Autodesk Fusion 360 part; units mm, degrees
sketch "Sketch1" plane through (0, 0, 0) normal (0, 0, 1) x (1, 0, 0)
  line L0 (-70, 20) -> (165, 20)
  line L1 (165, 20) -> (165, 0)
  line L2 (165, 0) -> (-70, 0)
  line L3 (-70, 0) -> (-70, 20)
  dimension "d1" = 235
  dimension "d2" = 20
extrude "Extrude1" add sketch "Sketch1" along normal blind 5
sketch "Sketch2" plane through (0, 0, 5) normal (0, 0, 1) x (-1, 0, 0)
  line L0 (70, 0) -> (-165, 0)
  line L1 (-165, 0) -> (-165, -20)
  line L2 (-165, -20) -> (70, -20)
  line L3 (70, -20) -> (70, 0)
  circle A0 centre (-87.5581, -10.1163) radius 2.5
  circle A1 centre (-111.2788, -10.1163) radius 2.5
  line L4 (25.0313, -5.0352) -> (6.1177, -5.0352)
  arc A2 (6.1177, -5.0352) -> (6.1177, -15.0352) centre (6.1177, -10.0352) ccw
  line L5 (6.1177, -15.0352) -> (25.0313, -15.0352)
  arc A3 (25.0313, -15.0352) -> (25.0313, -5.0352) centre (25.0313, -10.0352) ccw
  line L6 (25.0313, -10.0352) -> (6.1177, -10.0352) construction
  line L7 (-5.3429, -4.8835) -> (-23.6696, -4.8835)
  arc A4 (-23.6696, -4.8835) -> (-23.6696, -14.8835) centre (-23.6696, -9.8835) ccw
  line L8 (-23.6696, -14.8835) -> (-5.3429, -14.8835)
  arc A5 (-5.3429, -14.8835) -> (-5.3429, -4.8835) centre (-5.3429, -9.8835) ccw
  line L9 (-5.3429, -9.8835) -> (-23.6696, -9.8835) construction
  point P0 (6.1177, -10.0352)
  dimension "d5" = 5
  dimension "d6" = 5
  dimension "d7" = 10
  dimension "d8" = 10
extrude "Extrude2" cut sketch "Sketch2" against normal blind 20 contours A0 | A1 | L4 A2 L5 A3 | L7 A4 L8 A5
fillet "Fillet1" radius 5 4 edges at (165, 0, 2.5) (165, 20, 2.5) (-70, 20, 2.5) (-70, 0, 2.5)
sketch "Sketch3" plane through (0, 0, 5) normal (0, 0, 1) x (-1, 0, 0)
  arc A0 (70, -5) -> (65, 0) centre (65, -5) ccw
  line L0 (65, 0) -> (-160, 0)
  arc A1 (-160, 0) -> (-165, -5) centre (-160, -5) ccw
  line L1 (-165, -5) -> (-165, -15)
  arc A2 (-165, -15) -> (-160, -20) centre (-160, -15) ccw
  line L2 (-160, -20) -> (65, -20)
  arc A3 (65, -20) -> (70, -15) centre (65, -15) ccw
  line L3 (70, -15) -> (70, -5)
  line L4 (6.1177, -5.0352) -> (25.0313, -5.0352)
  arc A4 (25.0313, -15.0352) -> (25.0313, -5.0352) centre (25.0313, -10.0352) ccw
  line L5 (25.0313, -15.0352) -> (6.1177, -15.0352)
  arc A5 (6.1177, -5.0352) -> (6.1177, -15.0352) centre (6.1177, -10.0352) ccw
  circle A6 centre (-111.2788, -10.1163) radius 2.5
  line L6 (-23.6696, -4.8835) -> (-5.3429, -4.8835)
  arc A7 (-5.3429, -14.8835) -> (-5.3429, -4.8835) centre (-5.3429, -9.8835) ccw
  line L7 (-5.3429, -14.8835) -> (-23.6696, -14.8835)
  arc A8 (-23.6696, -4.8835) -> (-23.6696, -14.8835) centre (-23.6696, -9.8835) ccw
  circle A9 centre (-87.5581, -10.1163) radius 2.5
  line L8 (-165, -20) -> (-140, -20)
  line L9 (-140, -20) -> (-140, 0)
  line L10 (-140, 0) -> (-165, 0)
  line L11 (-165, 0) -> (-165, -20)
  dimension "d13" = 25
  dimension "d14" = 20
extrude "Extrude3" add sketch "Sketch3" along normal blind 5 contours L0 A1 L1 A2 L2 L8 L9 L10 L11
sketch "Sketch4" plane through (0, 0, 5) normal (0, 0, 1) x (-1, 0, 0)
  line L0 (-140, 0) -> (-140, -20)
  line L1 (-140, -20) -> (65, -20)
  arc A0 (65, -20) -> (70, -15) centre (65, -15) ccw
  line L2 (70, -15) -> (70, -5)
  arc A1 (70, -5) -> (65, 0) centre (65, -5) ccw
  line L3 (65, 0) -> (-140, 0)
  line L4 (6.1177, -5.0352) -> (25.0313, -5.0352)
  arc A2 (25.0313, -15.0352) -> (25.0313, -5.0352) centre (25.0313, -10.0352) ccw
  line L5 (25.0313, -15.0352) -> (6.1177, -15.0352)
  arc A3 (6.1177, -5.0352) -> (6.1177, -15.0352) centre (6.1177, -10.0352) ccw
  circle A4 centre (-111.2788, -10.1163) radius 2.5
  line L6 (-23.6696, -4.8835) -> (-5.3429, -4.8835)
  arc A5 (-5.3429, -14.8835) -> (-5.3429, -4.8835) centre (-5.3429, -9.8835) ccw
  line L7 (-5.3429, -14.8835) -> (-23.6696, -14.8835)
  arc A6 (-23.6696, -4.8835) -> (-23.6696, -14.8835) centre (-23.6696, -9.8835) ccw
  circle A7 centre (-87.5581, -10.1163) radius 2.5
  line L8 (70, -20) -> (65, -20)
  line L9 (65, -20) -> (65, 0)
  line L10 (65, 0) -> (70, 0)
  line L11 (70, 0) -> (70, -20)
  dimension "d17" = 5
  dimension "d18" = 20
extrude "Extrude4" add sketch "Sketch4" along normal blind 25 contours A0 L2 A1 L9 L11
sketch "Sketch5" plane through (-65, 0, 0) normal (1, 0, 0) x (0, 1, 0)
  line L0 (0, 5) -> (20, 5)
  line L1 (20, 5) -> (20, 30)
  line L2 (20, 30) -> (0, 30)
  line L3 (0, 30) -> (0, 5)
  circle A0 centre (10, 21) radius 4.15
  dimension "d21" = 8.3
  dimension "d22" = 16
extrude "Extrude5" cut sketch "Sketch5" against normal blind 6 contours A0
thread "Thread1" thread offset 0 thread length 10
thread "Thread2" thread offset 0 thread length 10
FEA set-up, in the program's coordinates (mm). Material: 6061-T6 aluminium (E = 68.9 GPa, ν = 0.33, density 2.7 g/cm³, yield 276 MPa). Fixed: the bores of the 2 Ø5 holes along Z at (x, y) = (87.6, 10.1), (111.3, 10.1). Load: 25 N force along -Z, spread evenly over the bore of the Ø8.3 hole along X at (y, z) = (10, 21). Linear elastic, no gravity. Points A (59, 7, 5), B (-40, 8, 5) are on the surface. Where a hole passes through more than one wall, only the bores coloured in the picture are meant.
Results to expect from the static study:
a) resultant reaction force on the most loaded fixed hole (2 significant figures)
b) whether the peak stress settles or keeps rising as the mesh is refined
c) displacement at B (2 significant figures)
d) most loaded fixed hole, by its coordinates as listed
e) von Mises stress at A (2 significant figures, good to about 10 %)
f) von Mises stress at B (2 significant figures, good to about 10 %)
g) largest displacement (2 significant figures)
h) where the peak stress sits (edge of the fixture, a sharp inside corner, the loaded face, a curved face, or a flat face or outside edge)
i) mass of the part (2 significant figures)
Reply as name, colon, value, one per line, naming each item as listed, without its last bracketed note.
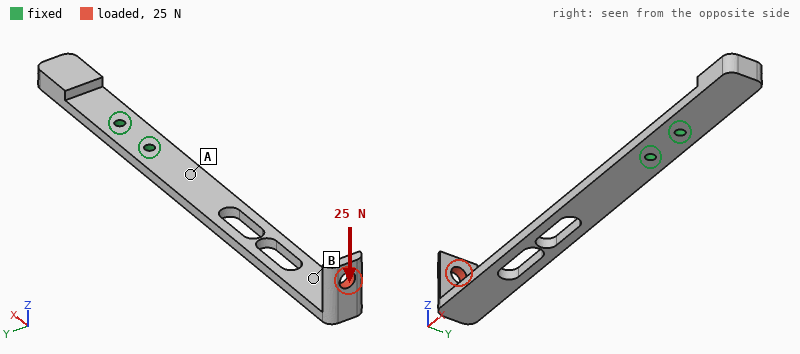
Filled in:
resultant reaction force on the most loaded fixed hole: 50 N
whether the peak stress settles or keeps rising as the mesh is refined: keeps rising
displacement at B: 1.9 mm
most loaded fixed hole, by its coordinates as listed: (87.6, 10.1)
von Mises stress at A: 38 MPa
von Mises stress at B: 8.2 MPa
largest displacement: 2.8 mm
where the peak stress sits: edge of the fixture
mass of the part: 67 g
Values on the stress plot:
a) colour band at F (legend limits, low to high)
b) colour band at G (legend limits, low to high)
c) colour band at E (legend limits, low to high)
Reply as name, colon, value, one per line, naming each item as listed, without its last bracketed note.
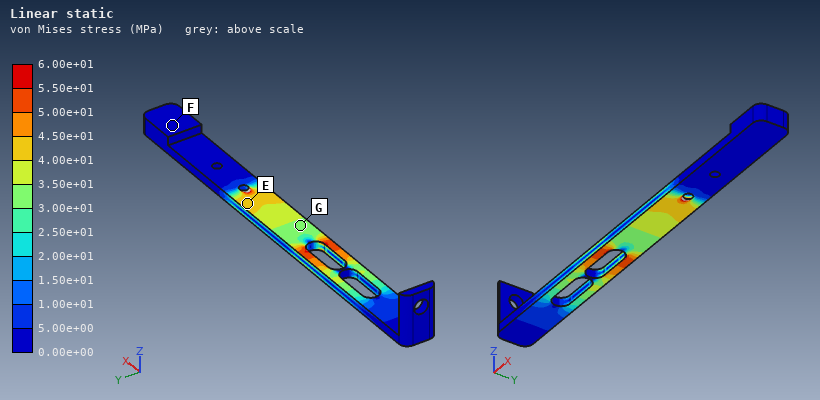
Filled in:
colour band at F: 0.00e+00 to 5.00e+00 MPa
colour band at G: 3.00e+01 to 3.50e+01 MPa
colour band at E: 4.00e+01 to 4.50e+01 MPa
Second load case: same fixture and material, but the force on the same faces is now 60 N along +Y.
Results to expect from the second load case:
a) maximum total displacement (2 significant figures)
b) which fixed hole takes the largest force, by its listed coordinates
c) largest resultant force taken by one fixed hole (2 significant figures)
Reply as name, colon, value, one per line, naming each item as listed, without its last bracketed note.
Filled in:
maximum total displacement: 0.91 mm
which fixed hole takes the largest force, by its listed coordinates: (87.6, 10.1)
largest resultant force taken by one fixed hole: 310 N
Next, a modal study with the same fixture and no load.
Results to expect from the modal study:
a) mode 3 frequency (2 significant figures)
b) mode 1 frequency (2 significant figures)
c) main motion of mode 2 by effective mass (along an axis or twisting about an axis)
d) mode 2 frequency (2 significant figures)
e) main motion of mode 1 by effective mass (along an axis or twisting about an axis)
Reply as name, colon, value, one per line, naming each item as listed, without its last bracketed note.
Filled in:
mode 3 frequency: 840 Hz
mode 1 frequency: 130 Hz
main motion of mode 2 by effective mass: along Y
mode 2 frequency: 460 Hz
main motion of mode 1 by effective mass: along Z
